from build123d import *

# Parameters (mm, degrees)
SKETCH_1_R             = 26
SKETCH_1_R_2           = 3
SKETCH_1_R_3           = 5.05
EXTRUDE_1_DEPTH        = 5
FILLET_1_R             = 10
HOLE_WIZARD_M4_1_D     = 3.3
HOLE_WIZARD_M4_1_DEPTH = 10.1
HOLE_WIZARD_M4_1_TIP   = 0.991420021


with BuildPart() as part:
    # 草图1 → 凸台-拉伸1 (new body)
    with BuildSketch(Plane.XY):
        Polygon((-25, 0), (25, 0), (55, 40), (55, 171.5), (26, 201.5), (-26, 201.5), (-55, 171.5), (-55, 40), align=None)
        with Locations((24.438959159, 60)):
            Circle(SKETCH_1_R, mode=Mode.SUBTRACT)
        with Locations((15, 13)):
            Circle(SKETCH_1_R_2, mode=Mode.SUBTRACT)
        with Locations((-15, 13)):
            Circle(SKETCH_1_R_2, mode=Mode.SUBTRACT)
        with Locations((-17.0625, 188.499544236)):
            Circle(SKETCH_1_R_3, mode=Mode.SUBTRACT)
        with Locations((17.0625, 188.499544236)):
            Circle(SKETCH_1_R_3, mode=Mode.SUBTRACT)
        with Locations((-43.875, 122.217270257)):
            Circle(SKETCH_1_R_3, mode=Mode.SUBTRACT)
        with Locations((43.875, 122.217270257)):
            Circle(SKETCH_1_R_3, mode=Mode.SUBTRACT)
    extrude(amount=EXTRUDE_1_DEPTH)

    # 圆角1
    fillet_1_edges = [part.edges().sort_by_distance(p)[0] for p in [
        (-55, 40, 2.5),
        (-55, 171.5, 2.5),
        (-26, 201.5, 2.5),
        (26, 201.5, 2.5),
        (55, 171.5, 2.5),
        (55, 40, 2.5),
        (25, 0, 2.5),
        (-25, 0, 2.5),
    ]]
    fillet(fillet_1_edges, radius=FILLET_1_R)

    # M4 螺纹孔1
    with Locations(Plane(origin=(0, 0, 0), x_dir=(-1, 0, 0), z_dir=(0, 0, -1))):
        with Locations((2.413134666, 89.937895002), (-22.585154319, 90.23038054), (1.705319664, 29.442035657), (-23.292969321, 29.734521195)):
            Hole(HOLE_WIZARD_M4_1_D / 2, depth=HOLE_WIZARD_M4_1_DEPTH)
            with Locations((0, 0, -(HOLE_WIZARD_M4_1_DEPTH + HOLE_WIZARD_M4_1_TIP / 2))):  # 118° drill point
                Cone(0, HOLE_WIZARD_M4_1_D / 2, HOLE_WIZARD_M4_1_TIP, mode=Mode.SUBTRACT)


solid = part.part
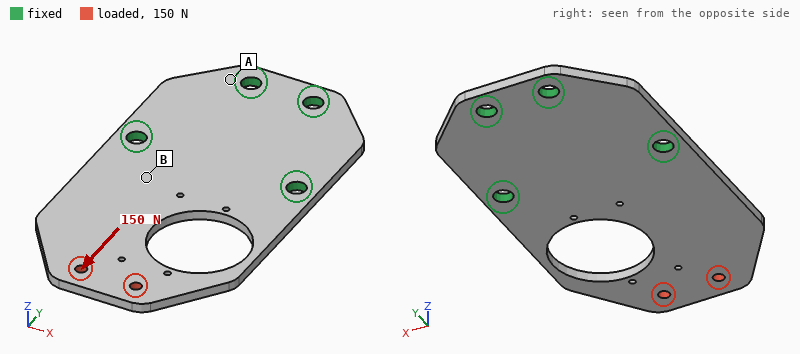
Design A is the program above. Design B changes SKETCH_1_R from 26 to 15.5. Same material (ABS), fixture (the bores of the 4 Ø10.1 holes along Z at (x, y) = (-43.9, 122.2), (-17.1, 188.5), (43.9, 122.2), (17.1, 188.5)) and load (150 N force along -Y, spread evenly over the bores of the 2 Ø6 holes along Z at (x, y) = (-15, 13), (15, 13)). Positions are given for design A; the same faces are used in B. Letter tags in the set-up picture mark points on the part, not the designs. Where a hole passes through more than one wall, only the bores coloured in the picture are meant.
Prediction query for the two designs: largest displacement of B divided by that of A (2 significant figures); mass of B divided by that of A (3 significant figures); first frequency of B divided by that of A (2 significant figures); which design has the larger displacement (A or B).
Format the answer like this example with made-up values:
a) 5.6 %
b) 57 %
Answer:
a) 0.40
b) 1.08
c) 1.0
d) A
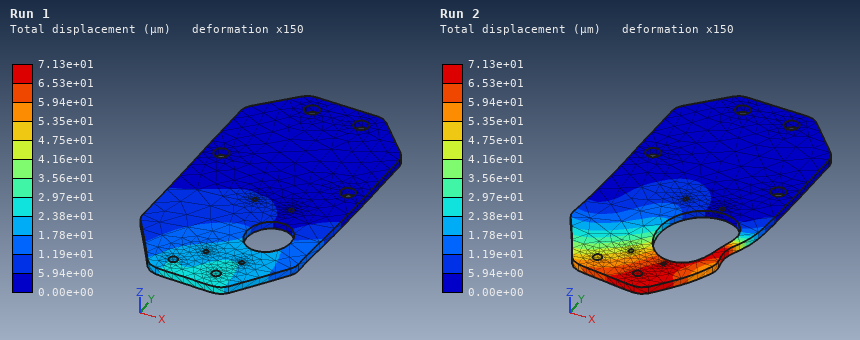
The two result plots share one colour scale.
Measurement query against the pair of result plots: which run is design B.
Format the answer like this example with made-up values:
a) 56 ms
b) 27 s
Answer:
a) Run 1
